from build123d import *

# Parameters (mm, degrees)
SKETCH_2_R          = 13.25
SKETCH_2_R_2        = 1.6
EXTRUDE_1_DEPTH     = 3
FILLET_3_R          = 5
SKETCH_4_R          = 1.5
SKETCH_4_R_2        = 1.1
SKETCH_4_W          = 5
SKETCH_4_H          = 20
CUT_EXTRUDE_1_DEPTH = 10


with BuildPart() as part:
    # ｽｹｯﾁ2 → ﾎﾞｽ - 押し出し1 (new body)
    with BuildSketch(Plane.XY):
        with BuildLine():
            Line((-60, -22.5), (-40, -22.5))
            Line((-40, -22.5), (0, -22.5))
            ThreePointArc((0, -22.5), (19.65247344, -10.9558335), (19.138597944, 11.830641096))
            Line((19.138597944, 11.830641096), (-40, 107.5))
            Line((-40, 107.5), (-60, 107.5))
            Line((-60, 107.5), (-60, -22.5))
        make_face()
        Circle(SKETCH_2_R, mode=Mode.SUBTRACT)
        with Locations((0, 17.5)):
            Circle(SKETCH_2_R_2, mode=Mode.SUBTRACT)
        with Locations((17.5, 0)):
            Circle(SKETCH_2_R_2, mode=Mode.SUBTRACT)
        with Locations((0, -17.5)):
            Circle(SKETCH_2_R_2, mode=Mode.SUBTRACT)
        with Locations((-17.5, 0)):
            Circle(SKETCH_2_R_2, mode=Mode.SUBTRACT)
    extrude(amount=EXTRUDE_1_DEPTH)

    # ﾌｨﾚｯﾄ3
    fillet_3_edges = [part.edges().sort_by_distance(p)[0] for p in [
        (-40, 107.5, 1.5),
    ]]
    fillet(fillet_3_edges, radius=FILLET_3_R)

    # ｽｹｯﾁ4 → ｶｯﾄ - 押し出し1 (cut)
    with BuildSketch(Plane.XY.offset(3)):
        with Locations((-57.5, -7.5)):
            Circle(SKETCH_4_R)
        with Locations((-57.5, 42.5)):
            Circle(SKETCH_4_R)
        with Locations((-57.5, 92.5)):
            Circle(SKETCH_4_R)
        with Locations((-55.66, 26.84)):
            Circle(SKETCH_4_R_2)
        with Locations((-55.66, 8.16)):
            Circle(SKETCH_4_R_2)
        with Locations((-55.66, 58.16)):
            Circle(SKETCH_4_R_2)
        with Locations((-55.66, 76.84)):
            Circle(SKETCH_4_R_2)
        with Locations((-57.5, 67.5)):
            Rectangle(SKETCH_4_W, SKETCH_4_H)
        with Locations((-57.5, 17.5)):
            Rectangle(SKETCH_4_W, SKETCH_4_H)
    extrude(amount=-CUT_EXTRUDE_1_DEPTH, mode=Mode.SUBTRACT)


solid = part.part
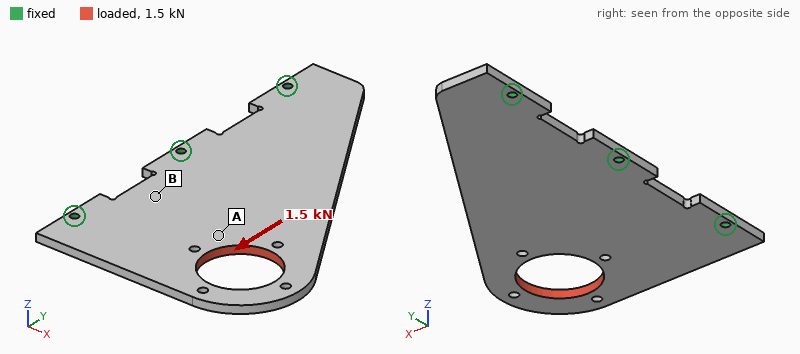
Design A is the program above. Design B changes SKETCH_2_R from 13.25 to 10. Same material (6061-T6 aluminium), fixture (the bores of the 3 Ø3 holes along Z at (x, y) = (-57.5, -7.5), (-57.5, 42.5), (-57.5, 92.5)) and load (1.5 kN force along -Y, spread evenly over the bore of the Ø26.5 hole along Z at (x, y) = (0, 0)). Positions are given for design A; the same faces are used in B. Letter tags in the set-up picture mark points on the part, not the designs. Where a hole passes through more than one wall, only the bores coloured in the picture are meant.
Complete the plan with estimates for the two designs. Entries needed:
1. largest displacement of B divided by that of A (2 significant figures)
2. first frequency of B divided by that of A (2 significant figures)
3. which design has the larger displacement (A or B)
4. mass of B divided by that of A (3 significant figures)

0.78
0.94
A
1.04
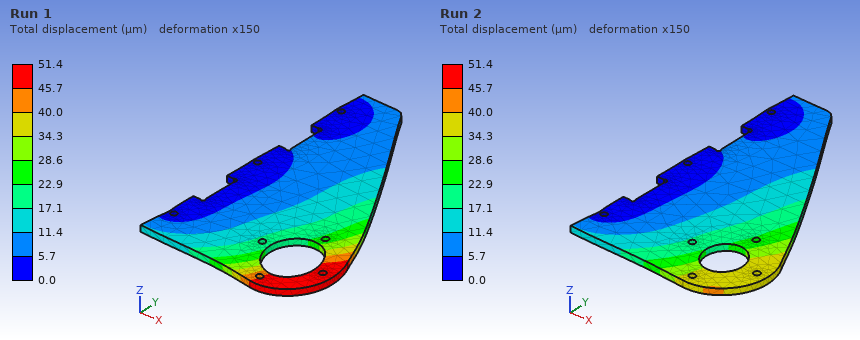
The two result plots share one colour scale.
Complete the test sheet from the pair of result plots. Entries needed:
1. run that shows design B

Run 2
